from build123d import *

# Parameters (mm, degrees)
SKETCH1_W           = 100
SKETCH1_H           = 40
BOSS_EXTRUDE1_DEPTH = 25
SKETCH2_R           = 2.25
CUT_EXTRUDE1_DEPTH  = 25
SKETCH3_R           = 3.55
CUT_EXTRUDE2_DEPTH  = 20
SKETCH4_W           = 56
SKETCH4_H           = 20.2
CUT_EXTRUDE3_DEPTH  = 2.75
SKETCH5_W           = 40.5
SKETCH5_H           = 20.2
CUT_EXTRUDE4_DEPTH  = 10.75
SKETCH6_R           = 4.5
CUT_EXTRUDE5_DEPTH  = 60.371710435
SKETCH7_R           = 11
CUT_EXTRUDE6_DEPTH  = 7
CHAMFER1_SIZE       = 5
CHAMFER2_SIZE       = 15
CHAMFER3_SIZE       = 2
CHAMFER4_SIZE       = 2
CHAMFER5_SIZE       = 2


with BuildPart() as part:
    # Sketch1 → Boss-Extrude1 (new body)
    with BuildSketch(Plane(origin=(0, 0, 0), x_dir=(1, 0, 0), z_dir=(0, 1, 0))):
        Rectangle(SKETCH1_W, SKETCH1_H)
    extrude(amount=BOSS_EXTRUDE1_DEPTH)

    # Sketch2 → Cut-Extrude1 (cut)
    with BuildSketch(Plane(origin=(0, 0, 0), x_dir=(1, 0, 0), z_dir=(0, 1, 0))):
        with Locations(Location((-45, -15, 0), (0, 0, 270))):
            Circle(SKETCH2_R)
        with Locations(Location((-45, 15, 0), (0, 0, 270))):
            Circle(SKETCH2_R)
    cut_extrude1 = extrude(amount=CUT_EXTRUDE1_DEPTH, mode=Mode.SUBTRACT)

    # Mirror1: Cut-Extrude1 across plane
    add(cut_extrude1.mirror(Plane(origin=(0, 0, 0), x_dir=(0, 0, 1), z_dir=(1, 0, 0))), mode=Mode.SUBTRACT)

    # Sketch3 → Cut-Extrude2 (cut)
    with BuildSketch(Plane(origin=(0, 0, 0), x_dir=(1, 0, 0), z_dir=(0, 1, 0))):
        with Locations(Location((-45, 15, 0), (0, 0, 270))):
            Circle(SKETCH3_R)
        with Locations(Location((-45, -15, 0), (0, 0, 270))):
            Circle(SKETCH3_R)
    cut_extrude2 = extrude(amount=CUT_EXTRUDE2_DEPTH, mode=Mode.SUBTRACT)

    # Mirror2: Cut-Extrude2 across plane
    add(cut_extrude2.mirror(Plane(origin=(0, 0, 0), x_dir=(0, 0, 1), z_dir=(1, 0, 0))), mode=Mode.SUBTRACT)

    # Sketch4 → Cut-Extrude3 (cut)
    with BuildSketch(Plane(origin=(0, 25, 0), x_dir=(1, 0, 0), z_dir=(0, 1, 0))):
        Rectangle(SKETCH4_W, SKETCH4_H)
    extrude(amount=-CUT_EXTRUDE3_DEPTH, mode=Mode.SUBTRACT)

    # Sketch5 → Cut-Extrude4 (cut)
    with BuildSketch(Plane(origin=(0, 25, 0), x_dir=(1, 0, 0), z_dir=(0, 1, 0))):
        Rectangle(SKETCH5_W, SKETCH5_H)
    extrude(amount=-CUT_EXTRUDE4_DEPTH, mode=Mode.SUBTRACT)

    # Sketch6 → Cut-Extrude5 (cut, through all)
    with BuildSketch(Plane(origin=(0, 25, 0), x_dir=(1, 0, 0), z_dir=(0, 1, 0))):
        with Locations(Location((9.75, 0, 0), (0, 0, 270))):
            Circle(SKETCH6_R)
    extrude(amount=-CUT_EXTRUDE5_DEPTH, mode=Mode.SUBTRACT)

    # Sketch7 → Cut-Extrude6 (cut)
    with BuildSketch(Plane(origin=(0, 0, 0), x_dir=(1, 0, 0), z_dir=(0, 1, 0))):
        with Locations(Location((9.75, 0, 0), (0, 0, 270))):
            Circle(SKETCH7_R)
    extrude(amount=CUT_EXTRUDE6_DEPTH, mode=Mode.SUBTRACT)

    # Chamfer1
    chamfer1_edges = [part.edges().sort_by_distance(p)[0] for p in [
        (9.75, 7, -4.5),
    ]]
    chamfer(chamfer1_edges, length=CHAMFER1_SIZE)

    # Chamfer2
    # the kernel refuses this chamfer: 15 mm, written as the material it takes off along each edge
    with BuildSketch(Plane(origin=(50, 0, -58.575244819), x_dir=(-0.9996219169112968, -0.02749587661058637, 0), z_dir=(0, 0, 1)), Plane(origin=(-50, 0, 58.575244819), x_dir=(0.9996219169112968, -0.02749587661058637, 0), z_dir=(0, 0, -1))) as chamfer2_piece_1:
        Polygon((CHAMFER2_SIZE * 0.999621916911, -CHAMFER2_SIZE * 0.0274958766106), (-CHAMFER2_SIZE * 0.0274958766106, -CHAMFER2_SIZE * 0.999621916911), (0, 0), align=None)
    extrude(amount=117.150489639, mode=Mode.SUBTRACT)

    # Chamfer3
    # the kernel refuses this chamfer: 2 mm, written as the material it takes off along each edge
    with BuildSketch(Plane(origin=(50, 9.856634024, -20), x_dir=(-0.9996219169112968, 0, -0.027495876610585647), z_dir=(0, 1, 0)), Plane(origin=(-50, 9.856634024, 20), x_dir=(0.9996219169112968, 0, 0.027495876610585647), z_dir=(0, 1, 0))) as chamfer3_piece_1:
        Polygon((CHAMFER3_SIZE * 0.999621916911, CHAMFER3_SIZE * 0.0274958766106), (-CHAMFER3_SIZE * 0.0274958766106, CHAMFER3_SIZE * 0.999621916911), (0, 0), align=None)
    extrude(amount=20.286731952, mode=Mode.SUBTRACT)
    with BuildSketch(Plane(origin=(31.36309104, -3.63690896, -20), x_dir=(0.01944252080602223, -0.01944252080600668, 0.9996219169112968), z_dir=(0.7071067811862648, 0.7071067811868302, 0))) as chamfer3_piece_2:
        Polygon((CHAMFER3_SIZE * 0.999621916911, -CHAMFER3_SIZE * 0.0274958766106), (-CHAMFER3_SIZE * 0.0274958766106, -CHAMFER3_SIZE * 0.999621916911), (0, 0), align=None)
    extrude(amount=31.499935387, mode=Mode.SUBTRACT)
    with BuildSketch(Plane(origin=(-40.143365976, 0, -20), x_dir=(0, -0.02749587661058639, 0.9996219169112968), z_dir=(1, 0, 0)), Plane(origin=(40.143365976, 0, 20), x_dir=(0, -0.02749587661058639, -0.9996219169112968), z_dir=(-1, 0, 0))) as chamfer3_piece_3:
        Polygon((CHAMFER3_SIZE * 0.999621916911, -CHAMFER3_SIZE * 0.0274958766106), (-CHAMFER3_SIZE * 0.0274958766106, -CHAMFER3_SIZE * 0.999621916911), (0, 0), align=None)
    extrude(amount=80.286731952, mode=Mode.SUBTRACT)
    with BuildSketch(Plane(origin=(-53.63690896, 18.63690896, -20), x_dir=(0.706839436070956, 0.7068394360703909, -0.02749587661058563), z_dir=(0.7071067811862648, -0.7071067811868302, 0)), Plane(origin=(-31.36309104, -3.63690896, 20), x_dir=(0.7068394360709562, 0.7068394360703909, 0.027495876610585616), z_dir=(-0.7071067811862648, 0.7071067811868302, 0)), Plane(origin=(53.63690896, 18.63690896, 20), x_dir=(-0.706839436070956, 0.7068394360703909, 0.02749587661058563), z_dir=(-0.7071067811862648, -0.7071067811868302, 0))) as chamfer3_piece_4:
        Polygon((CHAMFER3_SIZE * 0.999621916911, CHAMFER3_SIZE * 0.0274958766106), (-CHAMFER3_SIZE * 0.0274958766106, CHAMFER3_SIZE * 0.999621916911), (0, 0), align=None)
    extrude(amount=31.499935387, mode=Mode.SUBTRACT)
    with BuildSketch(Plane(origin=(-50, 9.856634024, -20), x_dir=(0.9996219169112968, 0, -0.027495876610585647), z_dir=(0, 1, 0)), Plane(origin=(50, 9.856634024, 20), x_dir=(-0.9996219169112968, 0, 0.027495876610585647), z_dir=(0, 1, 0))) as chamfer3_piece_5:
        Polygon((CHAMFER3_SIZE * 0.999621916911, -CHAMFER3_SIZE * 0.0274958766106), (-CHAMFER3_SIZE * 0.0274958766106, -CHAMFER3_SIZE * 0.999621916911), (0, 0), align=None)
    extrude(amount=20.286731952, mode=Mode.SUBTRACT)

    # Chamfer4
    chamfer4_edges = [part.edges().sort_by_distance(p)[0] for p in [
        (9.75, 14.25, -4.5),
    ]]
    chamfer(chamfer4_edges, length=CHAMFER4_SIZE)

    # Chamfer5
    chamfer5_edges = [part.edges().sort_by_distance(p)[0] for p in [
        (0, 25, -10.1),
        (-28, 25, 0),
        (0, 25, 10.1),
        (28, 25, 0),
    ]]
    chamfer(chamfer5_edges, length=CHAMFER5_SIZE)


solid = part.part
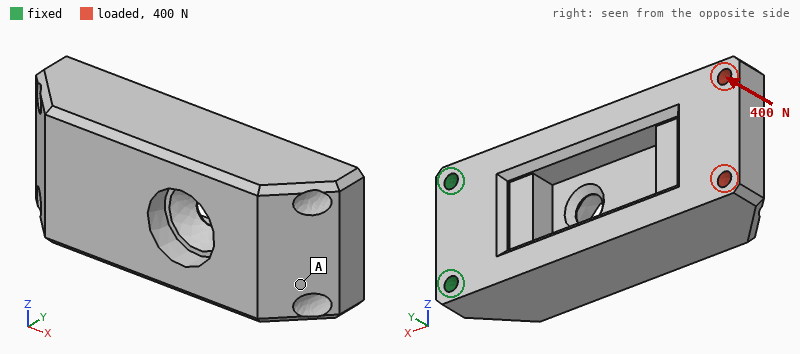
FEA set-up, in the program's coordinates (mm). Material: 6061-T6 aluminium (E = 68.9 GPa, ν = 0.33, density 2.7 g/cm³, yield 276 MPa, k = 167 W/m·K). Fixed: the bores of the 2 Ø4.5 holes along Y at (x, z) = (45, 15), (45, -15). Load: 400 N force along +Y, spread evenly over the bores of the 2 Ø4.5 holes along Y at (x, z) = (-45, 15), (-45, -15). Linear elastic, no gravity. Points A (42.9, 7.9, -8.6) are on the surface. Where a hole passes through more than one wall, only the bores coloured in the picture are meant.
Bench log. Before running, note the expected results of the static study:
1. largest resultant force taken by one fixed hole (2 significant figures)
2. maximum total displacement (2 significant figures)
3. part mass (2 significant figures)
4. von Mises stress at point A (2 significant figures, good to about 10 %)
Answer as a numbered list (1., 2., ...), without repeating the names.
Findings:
1. 220 N
2. 0.36 mm
3. 200 g
4. 19 MPa
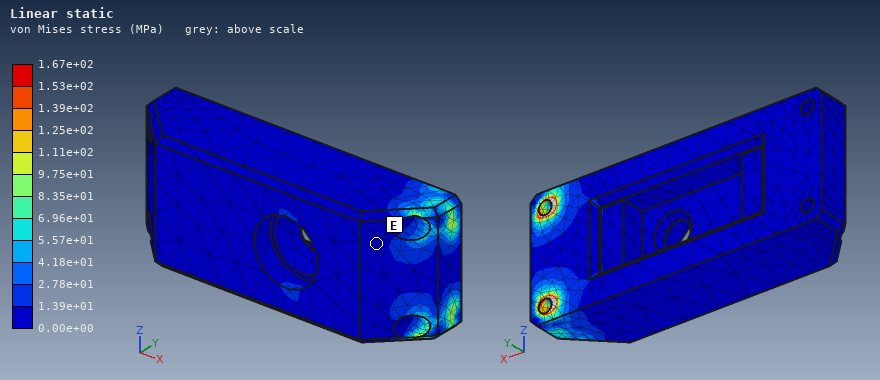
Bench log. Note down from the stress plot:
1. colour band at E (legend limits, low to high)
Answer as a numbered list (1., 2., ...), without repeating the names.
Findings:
1. 0.00e+00 to 1.39e+01 MPa
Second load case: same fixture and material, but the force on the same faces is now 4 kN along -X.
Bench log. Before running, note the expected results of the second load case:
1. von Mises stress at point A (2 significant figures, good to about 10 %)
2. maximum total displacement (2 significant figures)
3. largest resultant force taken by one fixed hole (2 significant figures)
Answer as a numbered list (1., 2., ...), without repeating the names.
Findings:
1. 6.0 MPa
2. 0.10 mm
3. 2.0 kN
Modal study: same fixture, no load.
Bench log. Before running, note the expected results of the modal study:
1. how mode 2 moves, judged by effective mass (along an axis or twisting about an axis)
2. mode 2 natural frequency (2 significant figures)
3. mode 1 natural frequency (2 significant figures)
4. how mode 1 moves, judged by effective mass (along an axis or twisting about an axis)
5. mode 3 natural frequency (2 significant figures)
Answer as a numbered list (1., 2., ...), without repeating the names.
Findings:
1. along Z
2. 2200 Hz
3. 650 Hz
4. along Y
5. 4900 Hz
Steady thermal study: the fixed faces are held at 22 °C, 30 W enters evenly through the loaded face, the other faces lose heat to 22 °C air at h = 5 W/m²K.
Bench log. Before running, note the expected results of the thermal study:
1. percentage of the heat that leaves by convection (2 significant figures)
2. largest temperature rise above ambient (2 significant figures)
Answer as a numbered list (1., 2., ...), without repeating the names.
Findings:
1. 4.1 %
2. 34 K
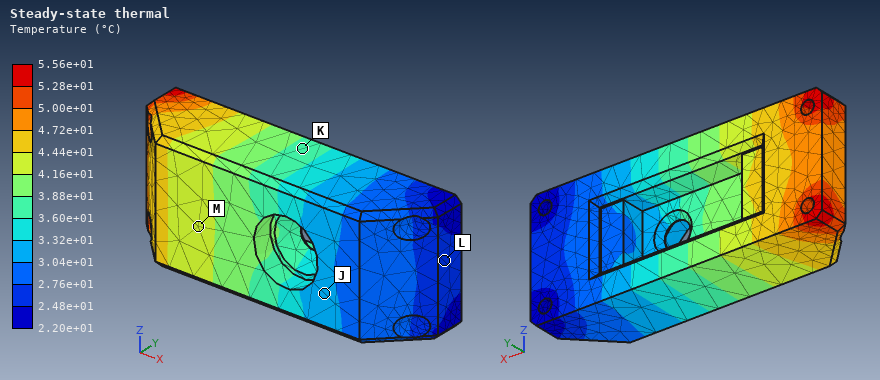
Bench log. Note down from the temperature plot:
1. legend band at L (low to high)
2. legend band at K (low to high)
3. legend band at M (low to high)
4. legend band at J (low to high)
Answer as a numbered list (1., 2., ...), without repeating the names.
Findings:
1. 2.48e+01 to 2.76e+01 °C
2. 3.60e+01 to 3.88e+01 °C
3. 4.16e+01 to 4.44e+01 °C
4. 3.04e+01 to 3.32e+01 °C
